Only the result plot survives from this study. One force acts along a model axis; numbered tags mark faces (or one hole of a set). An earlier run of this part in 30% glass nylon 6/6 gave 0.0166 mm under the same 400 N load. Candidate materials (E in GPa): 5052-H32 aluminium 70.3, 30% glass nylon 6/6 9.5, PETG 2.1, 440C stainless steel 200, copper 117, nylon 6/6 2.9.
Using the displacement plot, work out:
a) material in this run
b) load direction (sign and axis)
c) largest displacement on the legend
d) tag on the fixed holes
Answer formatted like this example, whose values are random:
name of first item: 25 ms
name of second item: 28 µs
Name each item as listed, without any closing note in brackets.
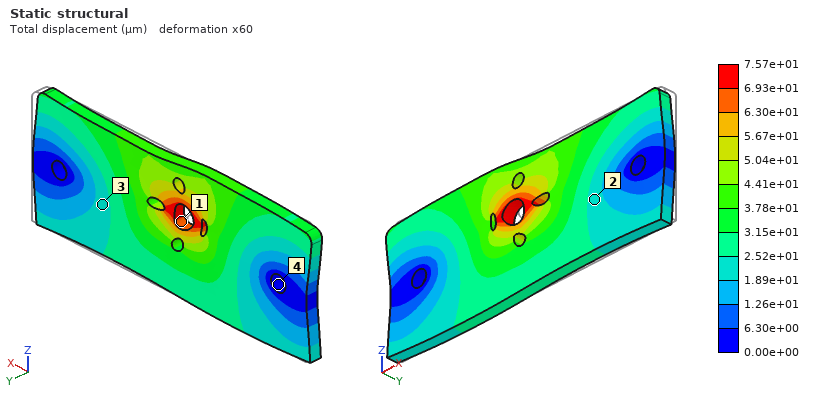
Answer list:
material in this run: PETG
load direction: -X
largest displacement on the legend: 7.57e+01 µm
tag on the fixed holes: 4
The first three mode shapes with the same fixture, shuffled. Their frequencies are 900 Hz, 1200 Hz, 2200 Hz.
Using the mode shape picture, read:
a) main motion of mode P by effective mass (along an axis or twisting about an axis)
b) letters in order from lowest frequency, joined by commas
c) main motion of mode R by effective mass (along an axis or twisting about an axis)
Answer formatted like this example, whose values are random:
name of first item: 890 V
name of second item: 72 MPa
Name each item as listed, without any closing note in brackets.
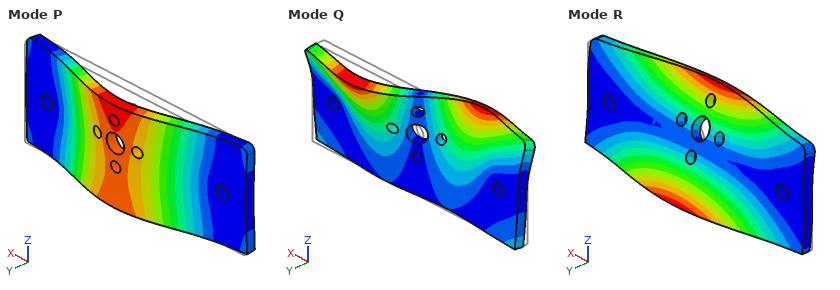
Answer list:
main motion of mode P by effective mass: along Y
letters in order from lowest frequency, joined by commas: P, R, Q
main motion of mode R by effective mass: twisting about X
